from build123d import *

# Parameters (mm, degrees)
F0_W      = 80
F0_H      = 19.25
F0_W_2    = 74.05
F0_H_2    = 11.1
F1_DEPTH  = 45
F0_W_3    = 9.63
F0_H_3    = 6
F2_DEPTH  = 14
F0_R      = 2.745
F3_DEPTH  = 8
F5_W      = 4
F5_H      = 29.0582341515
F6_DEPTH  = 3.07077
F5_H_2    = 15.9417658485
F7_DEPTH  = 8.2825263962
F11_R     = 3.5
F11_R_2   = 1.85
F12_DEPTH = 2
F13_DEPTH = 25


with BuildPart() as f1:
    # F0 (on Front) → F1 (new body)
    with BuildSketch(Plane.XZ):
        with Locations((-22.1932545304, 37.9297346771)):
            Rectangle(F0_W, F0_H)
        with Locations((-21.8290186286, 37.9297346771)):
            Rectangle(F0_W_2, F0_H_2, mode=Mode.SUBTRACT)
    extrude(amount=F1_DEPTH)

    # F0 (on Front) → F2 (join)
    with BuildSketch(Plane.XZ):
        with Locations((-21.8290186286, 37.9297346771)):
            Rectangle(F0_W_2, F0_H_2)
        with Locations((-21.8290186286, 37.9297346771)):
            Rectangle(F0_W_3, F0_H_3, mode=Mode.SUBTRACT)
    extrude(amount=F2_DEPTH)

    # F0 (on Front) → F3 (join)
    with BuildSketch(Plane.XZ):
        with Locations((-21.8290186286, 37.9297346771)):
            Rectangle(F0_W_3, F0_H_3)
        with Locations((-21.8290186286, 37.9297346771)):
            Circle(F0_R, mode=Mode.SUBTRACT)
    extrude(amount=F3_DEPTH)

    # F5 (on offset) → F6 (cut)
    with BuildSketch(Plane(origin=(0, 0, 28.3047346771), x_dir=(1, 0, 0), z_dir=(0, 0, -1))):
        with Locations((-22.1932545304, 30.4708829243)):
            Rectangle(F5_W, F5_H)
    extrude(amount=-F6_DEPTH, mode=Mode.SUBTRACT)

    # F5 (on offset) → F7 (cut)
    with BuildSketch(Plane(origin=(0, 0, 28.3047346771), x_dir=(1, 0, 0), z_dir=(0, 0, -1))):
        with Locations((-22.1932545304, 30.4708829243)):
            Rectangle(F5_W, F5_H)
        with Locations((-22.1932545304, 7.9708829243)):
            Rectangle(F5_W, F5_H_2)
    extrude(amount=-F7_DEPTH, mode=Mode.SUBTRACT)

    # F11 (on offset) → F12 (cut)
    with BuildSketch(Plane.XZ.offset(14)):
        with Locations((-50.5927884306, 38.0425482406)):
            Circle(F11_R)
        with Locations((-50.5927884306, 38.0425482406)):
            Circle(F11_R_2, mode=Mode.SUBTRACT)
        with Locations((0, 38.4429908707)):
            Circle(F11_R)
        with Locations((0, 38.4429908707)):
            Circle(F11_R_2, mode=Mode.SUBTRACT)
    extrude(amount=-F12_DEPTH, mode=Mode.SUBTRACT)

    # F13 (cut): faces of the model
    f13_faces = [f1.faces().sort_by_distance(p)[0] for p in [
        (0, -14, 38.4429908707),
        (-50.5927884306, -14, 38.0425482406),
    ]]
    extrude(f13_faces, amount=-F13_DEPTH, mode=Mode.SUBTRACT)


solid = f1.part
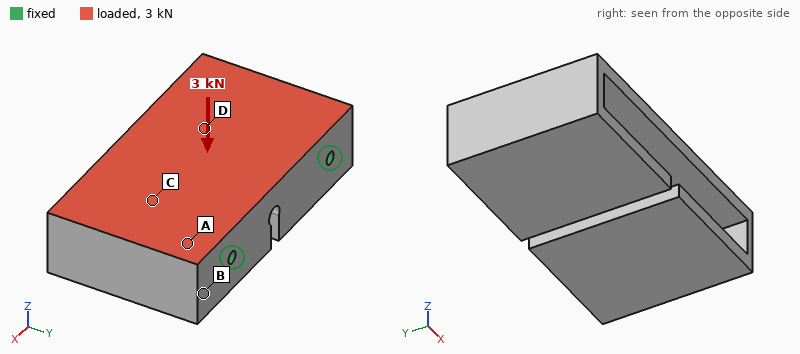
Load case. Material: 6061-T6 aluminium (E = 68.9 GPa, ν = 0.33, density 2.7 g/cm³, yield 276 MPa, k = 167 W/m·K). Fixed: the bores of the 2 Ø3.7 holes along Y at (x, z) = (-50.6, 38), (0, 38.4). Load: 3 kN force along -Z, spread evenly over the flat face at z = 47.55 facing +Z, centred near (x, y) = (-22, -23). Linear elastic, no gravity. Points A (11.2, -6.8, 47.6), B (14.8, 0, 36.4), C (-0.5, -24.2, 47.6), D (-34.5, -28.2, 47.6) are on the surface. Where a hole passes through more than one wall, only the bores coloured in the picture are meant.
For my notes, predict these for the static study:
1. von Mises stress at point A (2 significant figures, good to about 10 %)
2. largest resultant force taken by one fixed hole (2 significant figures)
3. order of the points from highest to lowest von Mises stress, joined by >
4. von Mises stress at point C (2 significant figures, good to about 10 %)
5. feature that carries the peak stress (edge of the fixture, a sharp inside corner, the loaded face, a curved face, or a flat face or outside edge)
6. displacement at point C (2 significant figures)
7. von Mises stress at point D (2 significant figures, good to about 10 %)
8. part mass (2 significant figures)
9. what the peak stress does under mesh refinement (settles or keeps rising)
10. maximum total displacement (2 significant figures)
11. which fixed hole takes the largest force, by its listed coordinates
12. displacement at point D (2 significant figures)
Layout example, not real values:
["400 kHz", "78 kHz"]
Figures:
["14 MPa", "1.8 kN", "C > D > A > B", "32 MPa", "edge of the fixture", "0.047 mm", "26 MPa", "110 g", "keeps rising", "0.19 mm", "(0, 38.4)", "0.076 mm"]
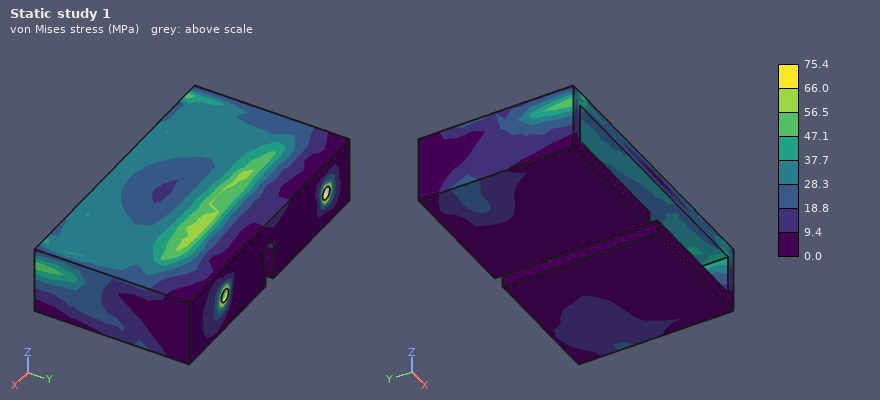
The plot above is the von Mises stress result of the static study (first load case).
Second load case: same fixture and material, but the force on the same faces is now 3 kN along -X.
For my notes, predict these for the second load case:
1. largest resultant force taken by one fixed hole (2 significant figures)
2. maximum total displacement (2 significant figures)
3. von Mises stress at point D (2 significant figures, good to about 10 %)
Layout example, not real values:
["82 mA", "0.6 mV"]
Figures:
["1.8 kN", "13 µm", "7.4 MPa"]
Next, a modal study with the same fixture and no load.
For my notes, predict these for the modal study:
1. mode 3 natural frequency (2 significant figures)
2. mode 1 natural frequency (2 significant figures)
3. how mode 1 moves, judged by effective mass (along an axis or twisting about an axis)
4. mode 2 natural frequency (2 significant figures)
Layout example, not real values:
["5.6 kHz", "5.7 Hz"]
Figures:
["4800 Hz", "3800 Hz", "along Z", "4200 Hz"]
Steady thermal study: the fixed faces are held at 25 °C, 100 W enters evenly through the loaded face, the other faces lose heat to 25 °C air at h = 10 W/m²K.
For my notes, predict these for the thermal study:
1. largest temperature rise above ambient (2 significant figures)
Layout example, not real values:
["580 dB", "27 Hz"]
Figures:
["29 K"]
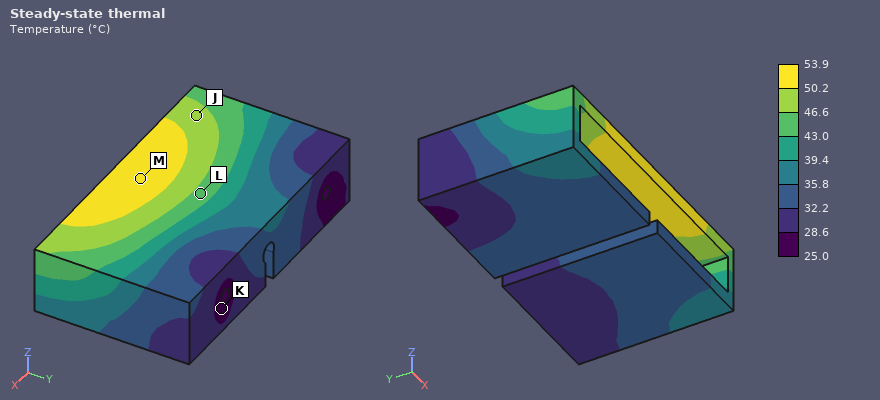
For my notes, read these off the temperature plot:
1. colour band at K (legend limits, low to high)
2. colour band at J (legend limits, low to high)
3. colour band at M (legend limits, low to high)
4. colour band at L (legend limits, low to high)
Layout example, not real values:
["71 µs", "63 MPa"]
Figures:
["25.0 to 28.6 °C", "46.6 to 50.2 °C", "50.2 to 53.9 °C", "43.0 to 46.6 °C"]
